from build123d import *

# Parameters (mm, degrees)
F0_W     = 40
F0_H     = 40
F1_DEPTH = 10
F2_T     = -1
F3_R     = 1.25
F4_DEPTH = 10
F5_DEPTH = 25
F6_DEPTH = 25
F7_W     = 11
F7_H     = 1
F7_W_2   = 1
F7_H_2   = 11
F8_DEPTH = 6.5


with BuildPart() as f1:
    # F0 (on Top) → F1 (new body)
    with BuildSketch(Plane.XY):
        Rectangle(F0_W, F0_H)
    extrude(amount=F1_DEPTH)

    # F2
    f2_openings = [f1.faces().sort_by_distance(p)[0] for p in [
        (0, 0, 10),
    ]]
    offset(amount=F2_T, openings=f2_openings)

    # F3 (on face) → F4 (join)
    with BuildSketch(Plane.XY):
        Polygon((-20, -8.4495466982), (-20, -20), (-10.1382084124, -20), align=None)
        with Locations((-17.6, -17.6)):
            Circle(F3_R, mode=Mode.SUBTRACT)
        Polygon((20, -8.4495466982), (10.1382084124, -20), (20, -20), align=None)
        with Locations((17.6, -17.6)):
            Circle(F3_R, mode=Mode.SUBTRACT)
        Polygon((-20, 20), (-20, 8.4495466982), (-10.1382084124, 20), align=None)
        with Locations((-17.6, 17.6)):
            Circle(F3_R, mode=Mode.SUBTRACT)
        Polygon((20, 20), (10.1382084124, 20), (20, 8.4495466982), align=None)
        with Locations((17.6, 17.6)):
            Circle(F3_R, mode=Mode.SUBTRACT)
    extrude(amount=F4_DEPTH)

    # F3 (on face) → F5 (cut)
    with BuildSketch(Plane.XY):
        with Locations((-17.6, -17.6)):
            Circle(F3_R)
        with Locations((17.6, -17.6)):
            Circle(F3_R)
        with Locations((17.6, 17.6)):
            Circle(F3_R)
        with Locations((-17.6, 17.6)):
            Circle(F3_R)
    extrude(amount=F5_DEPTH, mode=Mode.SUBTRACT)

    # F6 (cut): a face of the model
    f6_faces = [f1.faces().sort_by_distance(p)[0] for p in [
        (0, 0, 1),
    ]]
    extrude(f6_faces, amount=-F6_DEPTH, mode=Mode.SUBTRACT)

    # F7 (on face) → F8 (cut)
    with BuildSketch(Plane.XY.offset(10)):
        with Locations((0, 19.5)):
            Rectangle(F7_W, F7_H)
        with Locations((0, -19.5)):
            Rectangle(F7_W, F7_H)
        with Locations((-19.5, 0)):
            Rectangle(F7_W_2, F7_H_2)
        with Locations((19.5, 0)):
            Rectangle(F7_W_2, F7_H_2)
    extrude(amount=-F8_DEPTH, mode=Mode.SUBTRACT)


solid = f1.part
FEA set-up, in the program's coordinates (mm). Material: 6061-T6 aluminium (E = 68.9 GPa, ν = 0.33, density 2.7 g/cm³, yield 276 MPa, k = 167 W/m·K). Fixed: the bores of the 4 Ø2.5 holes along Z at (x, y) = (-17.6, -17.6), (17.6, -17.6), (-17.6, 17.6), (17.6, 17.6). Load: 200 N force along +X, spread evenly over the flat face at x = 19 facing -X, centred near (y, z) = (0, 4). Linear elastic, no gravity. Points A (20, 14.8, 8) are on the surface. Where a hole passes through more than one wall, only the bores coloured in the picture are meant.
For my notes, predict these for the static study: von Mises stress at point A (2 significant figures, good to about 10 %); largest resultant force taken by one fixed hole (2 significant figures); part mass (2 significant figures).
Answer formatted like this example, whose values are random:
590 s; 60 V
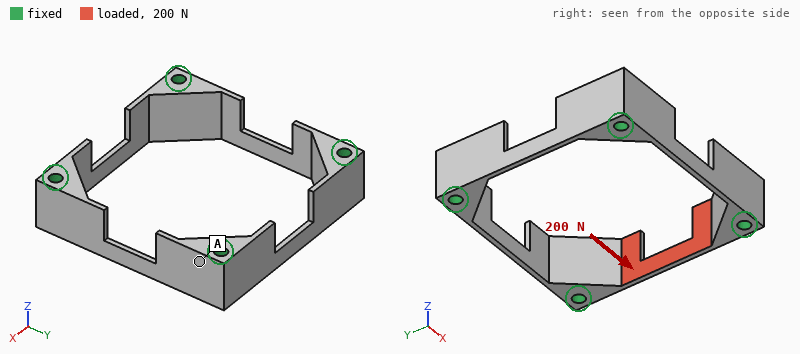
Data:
18 MPa; 120 N; 7.0 g
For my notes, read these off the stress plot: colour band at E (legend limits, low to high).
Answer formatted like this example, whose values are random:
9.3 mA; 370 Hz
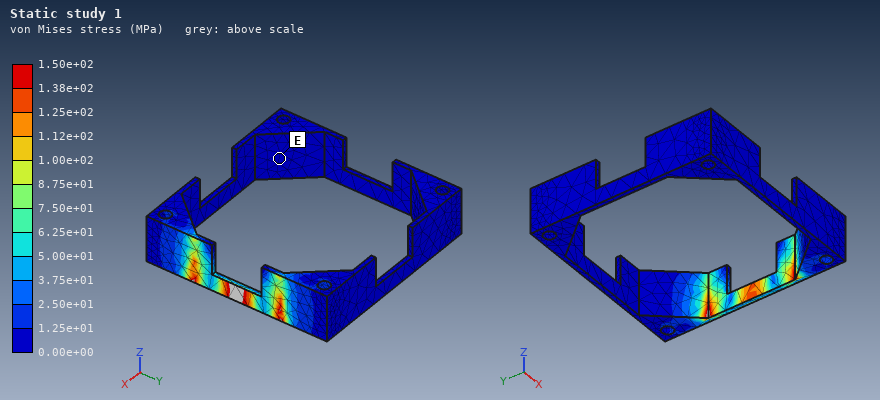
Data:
0.00e+00 to 1.25e+01 MPa
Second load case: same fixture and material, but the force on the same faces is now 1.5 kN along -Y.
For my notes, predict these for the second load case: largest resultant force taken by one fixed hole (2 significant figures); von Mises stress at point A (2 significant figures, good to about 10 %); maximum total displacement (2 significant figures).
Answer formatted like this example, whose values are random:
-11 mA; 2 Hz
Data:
750 N; 38 MPa; 20 µm
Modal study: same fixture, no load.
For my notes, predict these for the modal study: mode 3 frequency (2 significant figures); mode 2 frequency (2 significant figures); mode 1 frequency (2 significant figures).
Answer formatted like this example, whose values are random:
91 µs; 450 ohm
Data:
14 kHz; 12 kHz; 11 kHz
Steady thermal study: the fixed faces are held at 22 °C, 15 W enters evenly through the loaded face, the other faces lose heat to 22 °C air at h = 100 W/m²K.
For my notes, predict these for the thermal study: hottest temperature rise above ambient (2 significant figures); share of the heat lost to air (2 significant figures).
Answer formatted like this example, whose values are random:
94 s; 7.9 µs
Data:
40 K; 4.1 %
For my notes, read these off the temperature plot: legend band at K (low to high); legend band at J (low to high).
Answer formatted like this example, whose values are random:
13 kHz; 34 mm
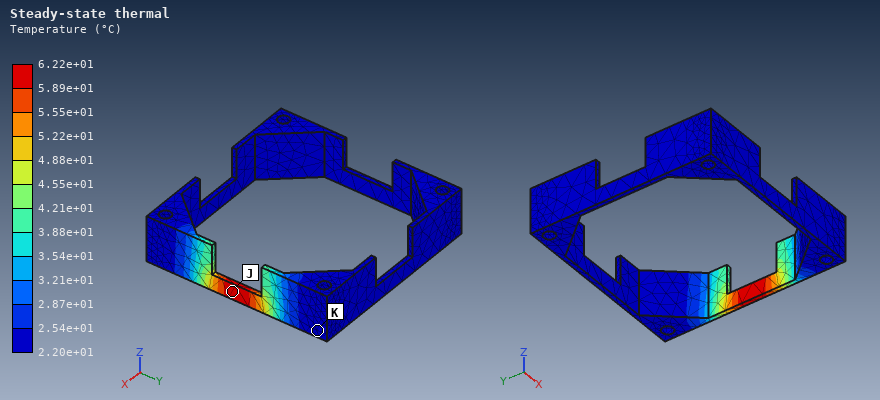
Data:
2.20e+01 to 2.54e+01 °C; 5.89e+01 to 6.22e+01 °C
